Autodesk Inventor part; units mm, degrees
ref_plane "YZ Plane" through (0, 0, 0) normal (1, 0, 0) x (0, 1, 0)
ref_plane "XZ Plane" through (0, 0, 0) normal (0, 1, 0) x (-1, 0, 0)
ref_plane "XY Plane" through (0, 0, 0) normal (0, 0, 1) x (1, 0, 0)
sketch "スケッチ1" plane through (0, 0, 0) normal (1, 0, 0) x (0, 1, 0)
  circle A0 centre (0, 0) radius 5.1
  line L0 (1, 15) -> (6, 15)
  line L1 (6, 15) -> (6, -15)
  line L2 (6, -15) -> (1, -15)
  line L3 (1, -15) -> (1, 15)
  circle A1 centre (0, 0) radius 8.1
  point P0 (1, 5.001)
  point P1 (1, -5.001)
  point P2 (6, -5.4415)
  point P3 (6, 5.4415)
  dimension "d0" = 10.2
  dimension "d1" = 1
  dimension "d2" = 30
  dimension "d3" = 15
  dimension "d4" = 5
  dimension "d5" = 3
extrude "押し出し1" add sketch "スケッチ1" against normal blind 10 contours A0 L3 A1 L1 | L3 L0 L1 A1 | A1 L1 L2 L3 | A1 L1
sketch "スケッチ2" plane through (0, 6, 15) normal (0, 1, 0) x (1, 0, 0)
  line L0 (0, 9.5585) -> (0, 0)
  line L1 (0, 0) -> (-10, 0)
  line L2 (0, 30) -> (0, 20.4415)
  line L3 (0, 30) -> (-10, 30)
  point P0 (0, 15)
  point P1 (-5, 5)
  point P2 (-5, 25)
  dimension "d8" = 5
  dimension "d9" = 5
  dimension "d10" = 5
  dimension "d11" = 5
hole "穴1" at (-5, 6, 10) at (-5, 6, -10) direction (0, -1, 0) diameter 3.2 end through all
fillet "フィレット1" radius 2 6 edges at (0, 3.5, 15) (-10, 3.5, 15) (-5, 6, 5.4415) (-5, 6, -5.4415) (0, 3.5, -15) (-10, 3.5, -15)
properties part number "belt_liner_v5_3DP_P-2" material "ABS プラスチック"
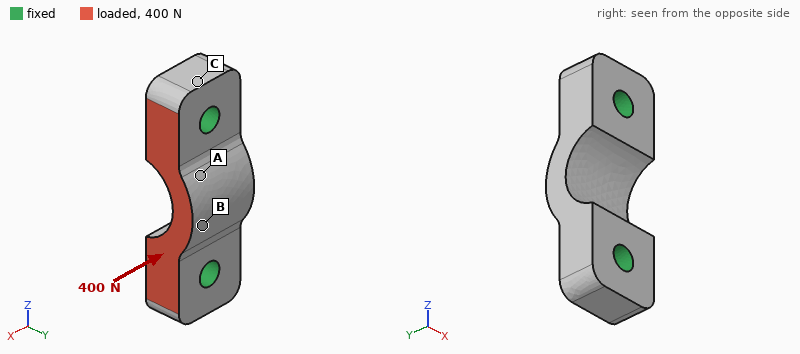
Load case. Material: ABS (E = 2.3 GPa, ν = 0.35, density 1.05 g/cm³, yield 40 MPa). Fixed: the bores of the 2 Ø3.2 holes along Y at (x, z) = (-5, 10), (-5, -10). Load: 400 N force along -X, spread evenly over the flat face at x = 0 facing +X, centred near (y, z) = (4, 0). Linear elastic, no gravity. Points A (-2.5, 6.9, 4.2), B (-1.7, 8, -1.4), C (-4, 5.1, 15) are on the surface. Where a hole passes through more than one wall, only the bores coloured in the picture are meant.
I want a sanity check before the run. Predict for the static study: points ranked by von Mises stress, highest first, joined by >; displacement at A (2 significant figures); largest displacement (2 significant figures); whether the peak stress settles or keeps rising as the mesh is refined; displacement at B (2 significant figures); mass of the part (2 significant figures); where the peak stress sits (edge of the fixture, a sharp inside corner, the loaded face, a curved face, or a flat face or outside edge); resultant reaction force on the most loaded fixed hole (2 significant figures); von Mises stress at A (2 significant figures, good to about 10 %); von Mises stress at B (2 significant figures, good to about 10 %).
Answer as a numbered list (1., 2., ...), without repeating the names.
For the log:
1. A > B > C
2. 42 µm
3. 68 µm
4. keeps rising
5. 59 µm
6. 1.3 g
7. edge of the fixture
8. 200 N
9. 6.0 MPa
10. 3.8 MPa
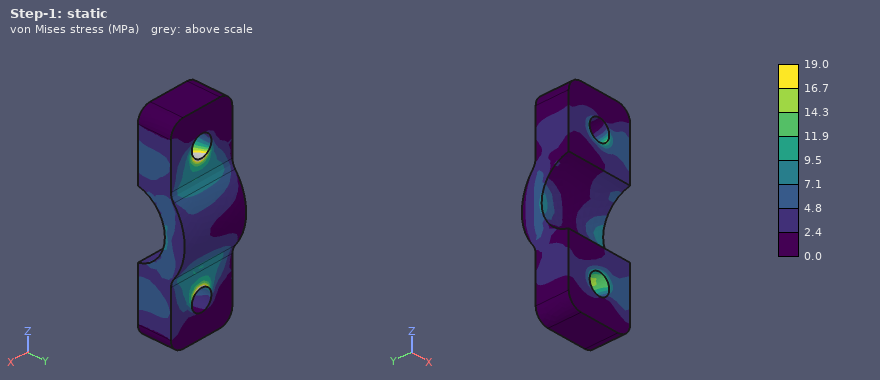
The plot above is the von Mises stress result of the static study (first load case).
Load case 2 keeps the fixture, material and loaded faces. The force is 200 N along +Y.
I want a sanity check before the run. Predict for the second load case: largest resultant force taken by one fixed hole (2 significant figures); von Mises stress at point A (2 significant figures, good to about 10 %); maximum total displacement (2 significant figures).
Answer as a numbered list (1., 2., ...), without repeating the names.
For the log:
1. 100 N
2. 4.7 MPa
3. 76 µm
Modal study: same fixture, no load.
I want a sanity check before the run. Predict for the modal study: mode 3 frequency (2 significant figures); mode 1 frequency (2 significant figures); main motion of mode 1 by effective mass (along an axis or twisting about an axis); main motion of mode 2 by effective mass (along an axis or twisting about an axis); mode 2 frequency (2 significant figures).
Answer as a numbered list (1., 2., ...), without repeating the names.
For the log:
1. 23 kHz
2. 14 kHz
3. along X
4. along Y
5. 18 kHz
